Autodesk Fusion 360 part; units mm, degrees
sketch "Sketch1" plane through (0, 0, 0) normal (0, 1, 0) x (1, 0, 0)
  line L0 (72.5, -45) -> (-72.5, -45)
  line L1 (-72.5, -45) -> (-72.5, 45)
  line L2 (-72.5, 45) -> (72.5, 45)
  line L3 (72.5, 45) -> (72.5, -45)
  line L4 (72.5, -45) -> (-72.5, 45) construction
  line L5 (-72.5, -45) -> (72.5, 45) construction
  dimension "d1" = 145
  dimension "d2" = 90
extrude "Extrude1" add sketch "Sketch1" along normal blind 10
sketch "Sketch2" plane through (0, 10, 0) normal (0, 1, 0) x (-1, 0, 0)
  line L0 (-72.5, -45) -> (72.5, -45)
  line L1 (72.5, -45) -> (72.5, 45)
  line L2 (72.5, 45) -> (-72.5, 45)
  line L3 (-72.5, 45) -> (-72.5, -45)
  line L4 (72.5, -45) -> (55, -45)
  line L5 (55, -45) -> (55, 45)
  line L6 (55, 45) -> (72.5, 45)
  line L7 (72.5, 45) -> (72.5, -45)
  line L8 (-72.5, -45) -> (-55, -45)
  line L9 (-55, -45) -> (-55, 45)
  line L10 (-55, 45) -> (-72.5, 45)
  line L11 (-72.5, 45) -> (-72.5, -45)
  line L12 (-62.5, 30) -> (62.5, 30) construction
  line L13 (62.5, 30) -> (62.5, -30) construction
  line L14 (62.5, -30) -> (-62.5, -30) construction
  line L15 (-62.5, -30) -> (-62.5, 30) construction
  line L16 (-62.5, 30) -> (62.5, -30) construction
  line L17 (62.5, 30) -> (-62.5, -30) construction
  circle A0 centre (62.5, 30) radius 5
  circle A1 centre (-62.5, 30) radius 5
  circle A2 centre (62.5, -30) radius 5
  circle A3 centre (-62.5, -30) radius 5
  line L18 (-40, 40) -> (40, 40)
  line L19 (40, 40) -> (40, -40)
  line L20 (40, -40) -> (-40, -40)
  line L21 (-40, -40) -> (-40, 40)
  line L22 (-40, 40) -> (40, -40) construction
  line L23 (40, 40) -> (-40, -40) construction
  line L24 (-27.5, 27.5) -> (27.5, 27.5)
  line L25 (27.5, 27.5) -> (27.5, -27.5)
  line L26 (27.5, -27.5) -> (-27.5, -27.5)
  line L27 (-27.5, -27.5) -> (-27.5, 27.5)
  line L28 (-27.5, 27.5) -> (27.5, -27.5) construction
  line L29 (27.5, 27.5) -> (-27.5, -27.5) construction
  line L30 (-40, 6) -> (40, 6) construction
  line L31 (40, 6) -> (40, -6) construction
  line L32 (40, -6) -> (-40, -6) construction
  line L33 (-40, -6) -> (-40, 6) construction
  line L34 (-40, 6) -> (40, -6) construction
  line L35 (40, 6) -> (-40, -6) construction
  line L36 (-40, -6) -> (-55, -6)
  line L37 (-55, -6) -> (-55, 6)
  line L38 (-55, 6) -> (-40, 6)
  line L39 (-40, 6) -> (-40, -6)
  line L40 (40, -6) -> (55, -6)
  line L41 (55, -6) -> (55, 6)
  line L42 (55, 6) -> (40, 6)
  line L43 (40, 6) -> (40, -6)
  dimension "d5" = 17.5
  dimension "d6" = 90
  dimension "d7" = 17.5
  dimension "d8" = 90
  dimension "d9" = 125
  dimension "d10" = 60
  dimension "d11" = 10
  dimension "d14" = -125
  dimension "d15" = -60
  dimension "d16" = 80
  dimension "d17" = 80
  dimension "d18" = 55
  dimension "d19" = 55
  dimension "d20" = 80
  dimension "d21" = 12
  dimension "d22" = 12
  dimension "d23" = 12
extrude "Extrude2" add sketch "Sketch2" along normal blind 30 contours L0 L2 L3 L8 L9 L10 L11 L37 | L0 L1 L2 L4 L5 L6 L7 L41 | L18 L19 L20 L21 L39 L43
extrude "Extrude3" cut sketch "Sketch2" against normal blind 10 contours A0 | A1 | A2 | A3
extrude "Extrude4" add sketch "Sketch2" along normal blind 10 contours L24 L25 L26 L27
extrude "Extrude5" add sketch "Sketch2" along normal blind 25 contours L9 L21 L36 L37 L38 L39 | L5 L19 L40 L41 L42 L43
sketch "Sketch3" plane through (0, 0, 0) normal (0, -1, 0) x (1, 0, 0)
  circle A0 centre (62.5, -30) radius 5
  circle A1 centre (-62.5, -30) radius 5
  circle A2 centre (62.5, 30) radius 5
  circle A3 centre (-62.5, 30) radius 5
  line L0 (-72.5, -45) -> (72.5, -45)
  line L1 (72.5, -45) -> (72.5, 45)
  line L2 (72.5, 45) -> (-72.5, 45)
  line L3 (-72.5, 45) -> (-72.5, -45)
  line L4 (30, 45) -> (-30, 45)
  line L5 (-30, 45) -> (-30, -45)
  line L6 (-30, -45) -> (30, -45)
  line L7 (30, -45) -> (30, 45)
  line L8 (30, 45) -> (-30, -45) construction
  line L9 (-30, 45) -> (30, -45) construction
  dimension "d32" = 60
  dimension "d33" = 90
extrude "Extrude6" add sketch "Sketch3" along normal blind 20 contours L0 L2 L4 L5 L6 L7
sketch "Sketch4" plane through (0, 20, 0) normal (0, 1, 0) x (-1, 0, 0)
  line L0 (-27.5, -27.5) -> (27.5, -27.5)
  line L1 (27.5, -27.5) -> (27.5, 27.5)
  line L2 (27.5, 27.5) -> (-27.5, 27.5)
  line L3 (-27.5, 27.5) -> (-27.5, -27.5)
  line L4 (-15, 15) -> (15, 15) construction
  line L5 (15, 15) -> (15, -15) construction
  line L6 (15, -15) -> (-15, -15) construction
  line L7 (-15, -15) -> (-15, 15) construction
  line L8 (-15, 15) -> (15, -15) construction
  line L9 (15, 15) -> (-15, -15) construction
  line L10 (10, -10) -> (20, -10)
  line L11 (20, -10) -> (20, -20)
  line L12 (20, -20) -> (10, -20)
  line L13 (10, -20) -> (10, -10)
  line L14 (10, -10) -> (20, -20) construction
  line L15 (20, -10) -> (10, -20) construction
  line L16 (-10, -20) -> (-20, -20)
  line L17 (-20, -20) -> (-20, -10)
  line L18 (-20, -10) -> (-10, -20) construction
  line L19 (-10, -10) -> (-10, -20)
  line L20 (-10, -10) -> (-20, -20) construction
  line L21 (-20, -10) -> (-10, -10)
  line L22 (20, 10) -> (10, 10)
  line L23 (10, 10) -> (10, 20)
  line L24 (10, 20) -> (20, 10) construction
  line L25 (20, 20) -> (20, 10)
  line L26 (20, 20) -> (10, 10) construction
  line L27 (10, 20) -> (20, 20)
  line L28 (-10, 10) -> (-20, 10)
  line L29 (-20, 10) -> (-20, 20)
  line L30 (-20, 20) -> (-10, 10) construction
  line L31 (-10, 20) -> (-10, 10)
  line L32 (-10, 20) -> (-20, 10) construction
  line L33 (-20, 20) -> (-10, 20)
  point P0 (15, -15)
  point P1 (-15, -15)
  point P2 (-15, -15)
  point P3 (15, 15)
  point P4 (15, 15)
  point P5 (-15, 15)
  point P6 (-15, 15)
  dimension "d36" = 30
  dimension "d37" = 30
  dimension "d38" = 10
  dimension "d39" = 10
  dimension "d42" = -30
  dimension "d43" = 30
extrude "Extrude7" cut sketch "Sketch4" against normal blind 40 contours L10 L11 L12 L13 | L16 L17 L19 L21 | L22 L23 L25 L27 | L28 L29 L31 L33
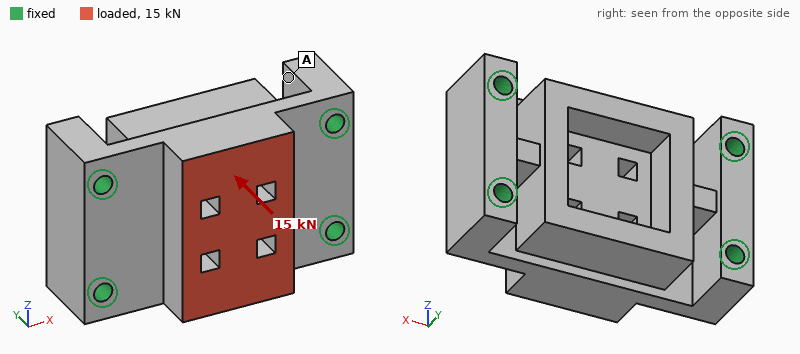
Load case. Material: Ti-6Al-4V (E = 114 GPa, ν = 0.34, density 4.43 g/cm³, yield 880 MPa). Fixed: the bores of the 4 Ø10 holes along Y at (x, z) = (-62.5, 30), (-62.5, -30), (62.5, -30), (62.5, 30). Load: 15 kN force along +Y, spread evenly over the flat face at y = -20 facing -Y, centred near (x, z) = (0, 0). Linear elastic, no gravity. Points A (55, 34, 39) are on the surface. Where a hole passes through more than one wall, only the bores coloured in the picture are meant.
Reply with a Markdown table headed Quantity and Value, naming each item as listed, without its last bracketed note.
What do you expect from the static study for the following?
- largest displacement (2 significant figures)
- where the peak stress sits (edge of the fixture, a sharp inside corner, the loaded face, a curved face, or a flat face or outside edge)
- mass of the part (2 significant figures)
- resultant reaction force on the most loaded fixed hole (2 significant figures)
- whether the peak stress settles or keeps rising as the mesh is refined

| Quantity | Value |
|---|---|
| largest displacement | 17 µm |
| where the peak stress sits | edge of the fixture |
| mass of the part | 2.0 kg |
| resultant reaction force on the most loaded fixed hole | 3.8 kN |
| whether the peak stress settles or keeps rising as the mesh is refined | keeps rising |
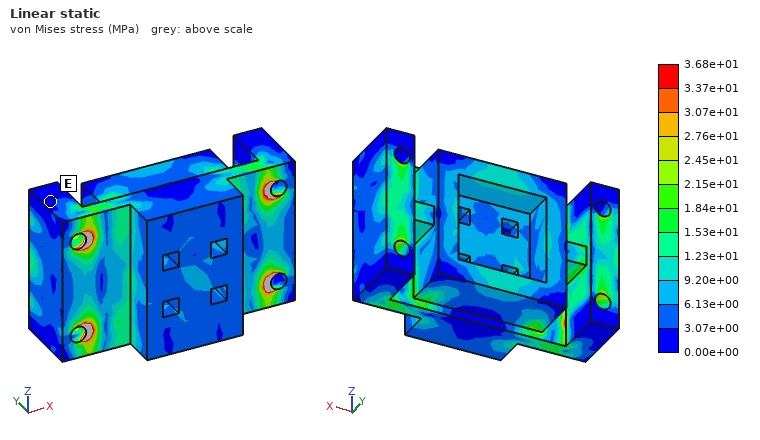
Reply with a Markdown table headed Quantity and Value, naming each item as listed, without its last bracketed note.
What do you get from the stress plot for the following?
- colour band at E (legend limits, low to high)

| Quantity | Value |
|---|---|
| colour band at E | 0.00e+00 to 3.07e+00 MPa |
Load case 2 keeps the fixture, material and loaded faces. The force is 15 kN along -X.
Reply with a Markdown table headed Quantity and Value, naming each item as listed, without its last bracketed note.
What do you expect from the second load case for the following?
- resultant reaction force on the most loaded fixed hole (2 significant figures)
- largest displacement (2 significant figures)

| Quantity | Value |
|---|---|
| resultant reaction force on the most loaded fixed hole | 4.3 kN |
| largest displacement | 12 µm |
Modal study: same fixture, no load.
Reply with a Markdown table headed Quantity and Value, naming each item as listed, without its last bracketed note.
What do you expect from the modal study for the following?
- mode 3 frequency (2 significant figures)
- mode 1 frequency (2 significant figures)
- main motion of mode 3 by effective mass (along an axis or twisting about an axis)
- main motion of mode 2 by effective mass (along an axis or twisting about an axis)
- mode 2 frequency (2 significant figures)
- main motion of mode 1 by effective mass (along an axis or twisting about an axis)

| Quantity | Value |
|---|---|
| mode 3 frequency | 6500 Hz |
| mode 1 frequency | 4100 Hz |
| main motion of mode 3 by effective mass | along Z |
| main motion of mode 2 by effective mass | along Y |
| mode 2 frequency | 4400 Hz |
| main motion of mode 1 by effective mass | twisting about X |
